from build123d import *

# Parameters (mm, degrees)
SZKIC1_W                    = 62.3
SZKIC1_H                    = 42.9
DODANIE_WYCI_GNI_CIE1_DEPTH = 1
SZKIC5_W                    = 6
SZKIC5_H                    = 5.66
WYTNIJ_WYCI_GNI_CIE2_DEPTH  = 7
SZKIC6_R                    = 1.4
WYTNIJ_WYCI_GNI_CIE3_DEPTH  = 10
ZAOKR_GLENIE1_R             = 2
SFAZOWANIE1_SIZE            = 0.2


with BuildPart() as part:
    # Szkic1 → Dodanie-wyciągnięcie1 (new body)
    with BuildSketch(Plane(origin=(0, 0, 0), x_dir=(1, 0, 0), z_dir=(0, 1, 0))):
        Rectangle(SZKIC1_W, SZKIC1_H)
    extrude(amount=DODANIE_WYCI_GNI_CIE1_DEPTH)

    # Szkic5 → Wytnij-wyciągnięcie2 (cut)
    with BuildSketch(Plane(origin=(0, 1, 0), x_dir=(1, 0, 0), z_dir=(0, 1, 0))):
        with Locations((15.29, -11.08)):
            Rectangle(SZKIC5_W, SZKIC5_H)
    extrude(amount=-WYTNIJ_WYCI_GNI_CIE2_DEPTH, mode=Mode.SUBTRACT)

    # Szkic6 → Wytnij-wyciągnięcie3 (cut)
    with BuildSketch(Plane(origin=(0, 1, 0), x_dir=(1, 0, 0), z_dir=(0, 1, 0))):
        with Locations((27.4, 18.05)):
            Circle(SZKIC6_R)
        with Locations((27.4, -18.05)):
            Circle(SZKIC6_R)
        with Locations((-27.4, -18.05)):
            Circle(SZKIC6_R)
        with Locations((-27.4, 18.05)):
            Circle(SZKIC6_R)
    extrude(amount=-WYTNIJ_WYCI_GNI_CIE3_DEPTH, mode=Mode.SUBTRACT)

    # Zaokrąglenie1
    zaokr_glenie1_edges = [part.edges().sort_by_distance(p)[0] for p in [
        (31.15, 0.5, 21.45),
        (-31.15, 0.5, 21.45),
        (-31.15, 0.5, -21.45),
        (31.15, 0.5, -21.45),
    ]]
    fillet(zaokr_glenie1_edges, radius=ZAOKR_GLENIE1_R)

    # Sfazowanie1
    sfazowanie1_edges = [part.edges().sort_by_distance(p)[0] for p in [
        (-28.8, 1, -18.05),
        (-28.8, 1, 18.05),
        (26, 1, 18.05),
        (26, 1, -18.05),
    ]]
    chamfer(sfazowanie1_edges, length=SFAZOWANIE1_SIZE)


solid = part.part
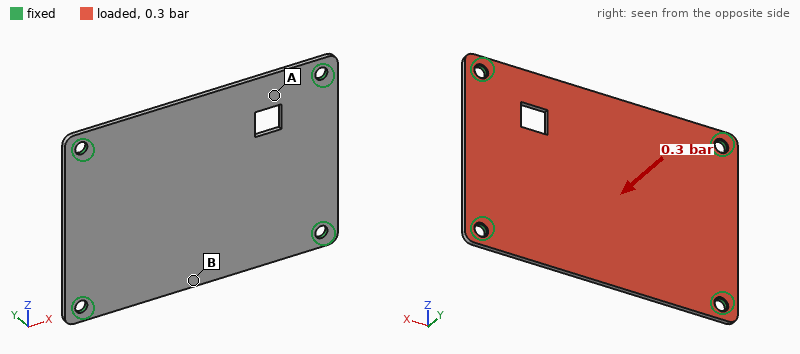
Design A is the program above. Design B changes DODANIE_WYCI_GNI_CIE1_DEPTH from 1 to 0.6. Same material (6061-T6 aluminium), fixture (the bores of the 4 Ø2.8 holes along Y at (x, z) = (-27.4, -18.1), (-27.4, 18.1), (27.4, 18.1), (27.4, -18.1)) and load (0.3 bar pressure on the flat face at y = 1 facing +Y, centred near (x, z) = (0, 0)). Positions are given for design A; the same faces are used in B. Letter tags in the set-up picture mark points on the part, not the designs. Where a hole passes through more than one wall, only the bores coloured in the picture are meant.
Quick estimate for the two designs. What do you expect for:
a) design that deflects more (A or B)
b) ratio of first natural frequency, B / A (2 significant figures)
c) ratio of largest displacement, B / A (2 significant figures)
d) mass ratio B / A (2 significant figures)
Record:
B
0.60
4.6
0.60
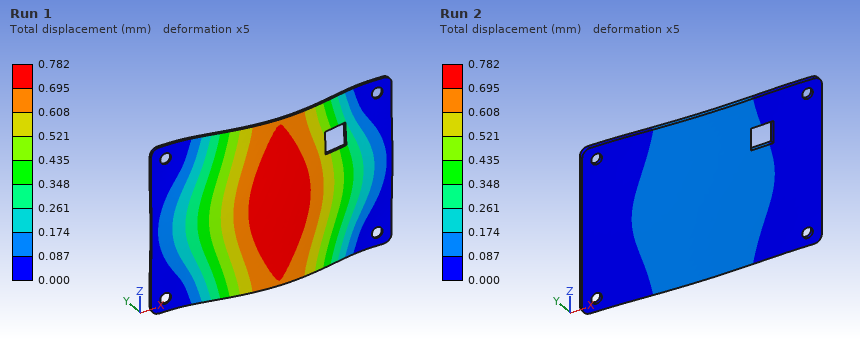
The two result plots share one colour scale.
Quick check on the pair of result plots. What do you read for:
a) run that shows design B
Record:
Run 1
